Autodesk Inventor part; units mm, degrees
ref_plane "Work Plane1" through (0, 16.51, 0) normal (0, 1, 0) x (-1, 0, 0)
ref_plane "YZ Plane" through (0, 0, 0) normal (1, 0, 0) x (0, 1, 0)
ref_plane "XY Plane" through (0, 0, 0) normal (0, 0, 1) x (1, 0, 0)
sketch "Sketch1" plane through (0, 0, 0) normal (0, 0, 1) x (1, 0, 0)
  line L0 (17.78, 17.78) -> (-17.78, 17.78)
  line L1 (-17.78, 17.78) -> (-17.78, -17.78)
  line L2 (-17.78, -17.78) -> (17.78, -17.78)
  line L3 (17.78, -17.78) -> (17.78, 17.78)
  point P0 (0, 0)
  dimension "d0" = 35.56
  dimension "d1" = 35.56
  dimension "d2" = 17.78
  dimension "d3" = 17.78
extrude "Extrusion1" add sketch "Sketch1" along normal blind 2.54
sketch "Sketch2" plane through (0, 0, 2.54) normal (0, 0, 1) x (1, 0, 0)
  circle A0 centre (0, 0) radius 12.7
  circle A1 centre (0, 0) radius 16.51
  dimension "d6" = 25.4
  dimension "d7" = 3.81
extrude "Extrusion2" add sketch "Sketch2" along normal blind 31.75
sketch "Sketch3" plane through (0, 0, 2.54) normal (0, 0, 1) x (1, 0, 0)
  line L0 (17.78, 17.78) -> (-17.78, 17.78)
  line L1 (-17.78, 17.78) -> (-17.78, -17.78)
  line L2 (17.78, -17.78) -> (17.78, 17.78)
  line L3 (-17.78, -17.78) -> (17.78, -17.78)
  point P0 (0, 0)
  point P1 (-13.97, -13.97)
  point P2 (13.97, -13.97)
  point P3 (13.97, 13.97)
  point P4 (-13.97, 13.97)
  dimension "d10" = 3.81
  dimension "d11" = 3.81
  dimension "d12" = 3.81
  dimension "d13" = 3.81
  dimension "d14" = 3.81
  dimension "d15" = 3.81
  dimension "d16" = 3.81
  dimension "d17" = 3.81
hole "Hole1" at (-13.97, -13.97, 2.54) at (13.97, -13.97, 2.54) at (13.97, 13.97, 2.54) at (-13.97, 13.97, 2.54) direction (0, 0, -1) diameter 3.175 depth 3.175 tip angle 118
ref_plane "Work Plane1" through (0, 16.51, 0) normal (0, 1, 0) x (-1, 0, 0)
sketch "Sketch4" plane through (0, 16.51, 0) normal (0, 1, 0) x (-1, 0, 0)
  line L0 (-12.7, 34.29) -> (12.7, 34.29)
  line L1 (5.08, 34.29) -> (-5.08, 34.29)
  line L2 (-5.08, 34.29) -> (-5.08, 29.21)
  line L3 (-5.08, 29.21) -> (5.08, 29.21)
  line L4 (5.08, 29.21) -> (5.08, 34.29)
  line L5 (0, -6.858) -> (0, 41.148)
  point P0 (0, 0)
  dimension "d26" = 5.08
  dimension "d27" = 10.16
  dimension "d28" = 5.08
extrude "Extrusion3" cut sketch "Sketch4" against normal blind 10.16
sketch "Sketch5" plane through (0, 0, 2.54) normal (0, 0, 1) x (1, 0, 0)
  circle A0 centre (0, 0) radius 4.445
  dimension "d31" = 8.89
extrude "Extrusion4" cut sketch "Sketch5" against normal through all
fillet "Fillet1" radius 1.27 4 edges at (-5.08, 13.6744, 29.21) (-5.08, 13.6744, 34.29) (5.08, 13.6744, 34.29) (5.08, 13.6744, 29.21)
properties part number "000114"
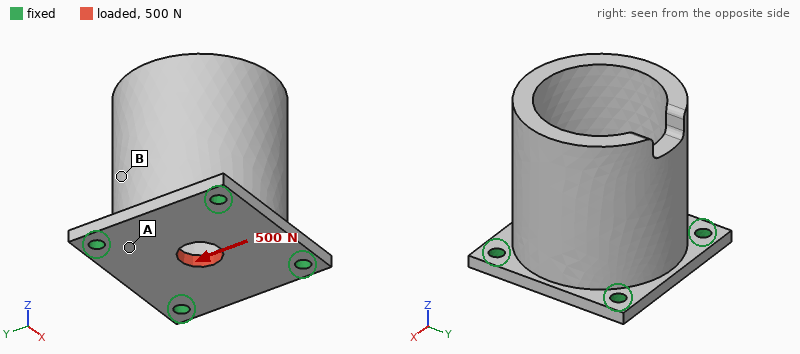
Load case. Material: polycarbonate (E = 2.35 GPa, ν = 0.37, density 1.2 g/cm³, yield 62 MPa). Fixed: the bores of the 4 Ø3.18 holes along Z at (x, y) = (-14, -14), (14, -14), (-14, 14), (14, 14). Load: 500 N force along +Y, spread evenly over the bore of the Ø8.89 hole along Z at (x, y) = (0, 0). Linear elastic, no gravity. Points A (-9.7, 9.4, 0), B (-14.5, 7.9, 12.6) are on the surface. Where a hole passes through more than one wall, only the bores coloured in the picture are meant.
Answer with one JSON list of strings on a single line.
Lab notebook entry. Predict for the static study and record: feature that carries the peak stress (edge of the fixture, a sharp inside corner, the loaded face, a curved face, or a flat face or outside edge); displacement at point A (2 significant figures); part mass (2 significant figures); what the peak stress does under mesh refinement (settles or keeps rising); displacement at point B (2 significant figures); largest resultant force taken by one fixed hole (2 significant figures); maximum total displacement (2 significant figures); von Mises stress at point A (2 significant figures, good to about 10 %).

["edge of the fixture", "18 µm", "17 g", "keeps rising", "13 µm", "140 N", "53 µm", "6.2 MPa"]
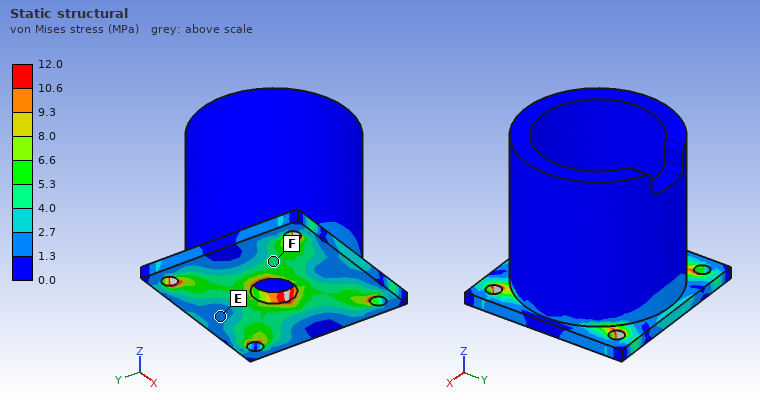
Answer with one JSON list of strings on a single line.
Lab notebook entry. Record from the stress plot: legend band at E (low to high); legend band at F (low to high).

["1.3 to 2.7 MPa", "4.0 to 5.3 MPa"]
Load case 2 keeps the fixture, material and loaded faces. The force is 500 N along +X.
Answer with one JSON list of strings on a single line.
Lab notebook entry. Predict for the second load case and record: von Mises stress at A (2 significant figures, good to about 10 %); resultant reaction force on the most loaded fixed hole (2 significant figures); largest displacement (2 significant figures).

["6.2 MPa", "140 N", "53 µm"]
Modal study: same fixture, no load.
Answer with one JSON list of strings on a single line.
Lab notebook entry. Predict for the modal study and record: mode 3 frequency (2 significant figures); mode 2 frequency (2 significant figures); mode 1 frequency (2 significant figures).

["3400 Hz", "2100 Hz", "2100 Hz"]
